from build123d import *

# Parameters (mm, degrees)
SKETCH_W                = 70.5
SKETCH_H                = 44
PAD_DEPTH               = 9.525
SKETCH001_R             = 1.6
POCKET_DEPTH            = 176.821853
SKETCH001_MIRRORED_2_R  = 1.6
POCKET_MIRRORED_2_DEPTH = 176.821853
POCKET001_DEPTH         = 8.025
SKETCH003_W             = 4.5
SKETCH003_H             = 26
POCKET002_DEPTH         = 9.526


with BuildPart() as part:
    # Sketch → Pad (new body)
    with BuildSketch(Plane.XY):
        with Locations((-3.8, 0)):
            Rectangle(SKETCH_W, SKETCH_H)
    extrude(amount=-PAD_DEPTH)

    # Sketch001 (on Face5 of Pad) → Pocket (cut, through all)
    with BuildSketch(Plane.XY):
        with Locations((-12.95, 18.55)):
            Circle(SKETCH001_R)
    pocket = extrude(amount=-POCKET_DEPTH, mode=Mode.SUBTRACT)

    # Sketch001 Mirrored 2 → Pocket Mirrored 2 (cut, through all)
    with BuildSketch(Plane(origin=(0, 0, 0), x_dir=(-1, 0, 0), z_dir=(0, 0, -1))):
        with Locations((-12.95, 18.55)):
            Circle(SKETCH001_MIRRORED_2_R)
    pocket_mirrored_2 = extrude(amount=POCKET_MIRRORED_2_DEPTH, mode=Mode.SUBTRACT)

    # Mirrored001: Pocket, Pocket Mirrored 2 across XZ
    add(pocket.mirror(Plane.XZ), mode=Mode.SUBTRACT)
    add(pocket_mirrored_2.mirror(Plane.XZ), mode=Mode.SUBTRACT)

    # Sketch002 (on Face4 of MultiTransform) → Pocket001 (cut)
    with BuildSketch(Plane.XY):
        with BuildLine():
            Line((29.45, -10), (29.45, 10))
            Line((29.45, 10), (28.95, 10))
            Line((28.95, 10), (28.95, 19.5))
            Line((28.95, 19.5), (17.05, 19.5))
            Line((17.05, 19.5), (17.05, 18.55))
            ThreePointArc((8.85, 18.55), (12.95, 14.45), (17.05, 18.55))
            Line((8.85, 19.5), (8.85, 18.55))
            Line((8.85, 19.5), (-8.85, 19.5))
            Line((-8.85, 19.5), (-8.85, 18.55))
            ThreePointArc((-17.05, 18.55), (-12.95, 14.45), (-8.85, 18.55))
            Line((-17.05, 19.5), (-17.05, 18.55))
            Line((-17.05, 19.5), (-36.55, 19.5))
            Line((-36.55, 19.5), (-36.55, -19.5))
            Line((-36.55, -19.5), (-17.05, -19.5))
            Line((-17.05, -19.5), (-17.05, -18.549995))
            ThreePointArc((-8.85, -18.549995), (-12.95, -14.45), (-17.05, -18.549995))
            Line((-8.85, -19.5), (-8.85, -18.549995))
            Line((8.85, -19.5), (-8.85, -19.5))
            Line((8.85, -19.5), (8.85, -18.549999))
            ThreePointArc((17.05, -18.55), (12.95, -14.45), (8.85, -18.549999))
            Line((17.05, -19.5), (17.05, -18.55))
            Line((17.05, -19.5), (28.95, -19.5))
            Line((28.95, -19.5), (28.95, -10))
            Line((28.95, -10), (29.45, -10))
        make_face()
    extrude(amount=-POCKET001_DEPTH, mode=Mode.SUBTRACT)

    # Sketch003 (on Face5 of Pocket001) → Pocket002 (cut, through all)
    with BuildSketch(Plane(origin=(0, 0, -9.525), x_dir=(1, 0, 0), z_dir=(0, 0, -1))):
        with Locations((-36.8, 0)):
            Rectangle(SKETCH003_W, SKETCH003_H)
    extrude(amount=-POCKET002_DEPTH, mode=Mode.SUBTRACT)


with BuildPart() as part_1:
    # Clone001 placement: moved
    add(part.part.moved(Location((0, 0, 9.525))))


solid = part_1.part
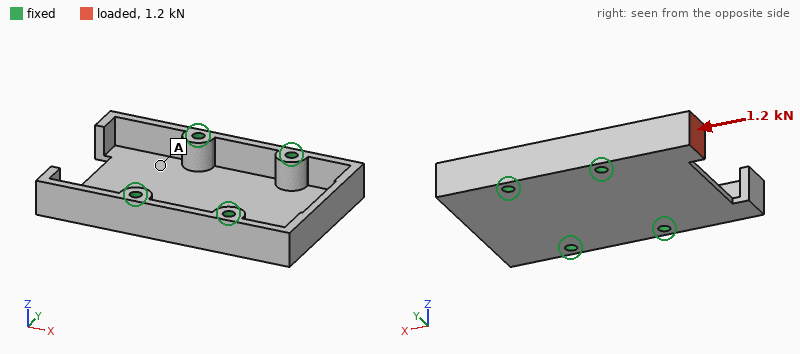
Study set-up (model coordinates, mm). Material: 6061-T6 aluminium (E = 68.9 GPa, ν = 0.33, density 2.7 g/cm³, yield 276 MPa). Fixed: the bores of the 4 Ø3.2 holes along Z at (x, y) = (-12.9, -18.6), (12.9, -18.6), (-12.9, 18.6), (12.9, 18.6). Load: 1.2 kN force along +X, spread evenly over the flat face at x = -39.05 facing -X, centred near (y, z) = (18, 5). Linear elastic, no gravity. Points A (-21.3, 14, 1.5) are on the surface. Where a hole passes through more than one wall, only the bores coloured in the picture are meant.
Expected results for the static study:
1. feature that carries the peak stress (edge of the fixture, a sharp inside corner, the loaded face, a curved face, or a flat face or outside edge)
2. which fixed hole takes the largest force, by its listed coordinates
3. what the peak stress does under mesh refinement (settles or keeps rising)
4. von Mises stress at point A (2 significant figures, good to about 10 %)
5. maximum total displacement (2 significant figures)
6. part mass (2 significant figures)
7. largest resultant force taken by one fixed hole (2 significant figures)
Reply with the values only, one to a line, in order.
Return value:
a sharp inside corner
(-12.9, 18.6)
keeps rising
20 MPa
0.11 mm
24 g
1.1 kN
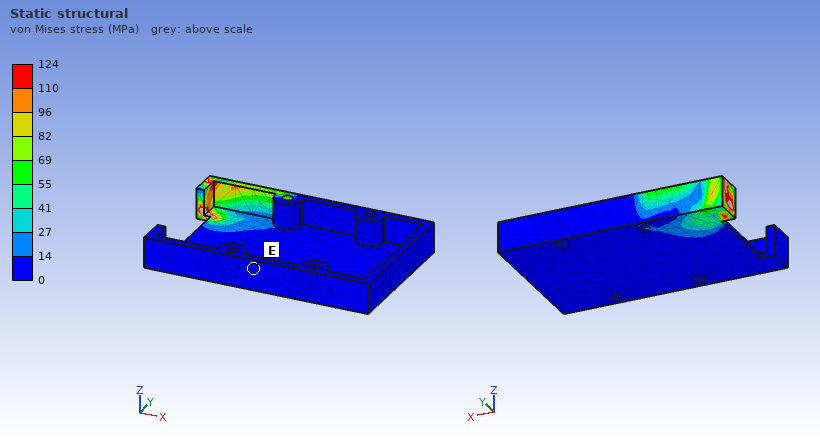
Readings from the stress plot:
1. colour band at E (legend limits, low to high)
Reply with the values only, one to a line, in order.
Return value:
0 to 14 MPa
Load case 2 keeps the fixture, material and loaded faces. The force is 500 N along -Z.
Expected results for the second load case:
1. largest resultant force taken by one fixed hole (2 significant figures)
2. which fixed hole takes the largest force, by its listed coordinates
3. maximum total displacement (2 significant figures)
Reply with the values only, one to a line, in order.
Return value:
530 N
(-12.9, 18.6)
0.29 mm
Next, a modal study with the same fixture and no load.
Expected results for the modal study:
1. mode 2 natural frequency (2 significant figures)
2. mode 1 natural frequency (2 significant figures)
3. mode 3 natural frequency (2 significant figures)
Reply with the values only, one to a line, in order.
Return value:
7300 Hz
4900 Hz
7600 Hz
